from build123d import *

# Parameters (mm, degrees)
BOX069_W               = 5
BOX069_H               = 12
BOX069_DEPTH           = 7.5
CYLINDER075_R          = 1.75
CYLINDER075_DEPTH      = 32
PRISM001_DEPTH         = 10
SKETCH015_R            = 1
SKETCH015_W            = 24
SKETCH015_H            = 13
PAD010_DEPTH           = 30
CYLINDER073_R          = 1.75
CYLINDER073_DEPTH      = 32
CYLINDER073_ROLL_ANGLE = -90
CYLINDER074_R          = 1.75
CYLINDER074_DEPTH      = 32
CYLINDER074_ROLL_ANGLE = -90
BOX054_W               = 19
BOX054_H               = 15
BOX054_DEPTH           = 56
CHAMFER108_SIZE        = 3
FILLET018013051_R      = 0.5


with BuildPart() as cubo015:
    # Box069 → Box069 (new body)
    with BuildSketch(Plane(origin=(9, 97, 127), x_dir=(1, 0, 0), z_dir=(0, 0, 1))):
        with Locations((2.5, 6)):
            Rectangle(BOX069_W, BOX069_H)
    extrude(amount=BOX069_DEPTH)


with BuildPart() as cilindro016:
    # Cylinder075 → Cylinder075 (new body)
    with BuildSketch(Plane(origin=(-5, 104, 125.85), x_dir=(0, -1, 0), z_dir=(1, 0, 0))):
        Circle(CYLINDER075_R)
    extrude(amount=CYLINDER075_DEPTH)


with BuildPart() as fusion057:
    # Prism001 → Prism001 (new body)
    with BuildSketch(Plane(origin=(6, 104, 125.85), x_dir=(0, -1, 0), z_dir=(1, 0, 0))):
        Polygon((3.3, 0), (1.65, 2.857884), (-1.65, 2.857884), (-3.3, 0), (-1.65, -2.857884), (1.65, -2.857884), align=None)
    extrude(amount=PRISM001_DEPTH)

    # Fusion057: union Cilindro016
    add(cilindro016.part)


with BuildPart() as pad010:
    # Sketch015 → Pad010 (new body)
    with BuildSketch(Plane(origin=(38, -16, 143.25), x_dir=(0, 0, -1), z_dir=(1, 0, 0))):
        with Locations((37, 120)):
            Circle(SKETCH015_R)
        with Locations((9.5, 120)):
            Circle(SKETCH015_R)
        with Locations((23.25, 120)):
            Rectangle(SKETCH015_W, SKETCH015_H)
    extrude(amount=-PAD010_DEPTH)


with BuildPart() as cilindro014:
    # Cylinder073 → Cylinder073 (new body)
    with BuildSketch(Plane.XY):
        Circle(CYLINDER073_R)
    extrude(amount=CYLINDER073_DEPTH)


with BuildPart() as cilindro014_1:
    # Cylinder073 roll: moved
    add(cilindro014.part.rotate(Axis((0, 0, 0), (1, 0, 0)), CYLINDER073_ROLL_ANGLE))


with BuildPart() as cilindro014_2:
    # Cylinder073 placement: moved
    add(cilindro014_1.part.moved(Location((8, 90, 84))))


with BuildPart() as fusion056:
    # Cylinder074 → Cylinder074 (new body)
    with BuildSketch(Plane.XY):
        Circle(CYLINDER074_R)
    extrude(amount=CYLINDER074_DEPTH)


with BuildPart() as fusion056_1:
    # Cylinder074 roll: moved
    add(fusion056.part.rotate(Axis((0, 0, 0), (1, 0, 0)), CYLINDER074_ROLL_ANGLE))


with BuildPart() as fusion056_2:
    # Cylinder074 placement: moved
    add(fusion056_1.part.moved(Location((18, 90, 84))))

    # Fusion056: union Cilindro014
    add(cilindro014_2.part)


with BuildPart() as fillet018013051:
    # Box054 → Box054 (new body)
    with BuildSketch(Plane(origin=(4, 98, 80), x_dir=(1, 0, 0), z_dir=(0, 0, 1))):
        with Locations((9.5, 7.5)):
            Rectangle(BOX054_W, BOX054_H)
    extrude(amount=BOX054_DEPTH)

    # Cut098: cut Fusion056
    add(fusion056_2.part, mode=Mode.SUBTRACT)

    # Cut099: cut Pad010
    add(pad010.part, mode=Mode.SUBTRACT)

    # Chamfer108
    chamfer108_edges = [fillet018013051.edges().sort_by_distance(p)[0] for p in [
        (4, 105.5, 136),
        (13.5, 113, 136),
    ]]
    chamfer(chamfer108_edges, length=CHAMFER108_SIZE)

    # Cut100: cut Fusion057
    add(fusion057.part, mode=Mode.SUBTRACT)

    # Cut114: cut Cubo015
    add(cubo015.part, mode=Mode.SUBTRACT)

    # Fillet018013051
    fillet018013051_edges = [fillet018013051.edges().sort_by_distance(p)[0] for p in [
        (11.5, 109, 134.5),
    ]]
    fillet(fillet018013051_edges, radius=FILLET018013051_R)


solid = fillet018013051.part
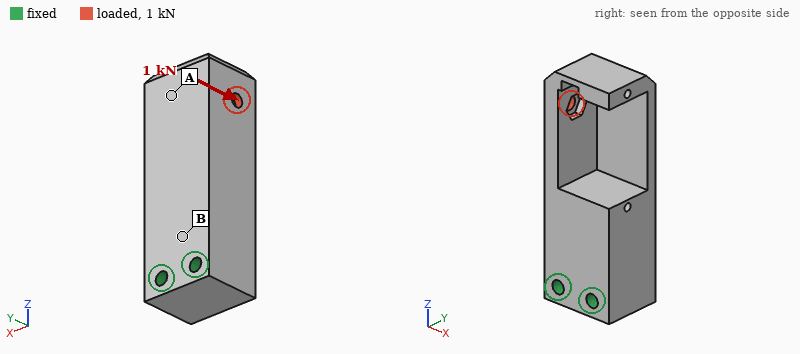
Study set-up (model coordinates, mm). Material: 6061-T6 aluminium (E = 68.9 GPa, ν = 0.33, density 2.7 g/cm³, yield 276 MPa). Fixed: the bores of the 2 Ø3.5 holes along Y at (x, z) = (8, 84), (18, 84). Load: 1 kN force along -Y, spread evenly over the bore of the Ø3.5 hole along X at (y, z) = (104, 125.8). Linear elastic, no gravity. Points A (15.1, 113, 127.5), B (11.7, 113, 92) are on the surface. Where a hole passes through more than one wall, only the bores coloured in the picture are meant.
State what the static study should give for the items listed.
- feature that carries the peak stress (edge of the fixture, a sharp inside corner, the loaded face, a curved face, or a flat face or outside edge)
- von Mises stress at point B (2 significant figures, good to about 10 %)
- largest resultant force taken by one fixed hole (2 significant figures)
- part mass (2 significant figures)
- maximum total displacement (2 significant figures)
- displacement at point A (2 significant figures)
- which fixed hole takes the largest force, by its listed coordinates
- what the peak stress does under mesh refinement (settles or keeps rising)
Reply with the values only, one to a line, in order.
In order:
a sharp inside corner
51 MPa
820 N
29 g
0.18 mm
0.12 mm
(8, 84)
keeps rising
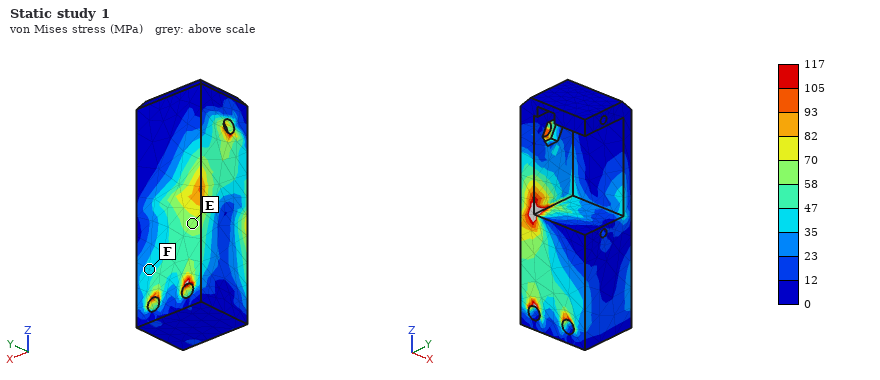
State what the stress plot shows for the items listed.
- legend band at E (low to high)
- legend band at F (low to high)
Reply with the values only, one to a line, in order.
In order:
58 to 70 MPa
35 to 47 MPa
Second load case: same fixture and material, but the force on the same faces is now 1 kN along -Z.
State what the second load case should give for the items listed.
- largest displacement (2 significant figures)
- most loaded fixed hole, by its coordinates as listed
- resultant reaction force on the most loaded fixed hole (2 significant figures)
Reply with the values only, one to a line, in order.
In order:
39 µm
(8, 84)
1.2 kN
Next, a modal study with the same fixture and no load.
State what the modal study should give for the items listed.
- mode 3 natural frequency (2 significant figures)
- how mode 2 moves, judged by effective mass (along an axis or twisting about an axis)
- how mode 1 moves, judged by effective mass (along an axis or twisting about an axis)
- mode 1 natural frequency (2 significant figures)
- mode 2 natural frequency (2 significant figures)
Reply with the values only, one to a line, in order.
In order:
9000 Hz
along X
along Y
4000 Hz
5100 Hz
